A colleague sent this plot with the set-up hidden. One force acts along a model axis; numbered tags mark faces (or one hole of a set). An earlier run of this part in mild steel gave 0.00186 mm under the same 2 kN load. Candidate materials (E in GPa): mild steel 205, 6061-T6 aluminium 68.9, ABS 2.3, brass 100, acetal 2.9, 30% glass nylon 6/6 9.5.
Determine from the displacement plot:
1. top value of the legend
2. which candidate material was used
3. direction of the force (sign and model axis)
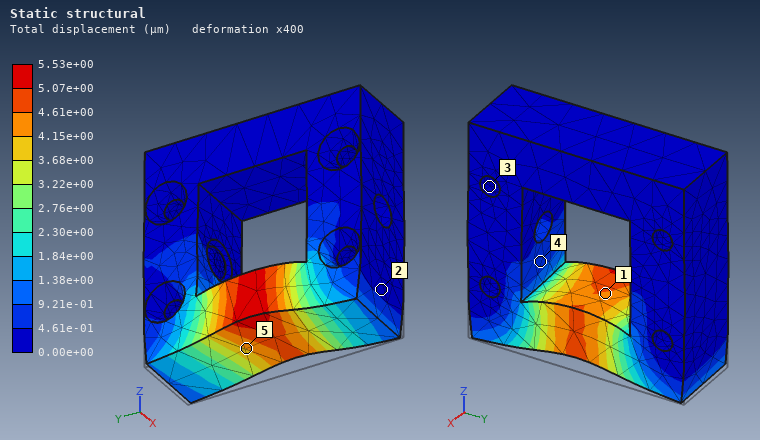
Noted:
5.53e+00 µm
6061-T6 aluminium
+Z
